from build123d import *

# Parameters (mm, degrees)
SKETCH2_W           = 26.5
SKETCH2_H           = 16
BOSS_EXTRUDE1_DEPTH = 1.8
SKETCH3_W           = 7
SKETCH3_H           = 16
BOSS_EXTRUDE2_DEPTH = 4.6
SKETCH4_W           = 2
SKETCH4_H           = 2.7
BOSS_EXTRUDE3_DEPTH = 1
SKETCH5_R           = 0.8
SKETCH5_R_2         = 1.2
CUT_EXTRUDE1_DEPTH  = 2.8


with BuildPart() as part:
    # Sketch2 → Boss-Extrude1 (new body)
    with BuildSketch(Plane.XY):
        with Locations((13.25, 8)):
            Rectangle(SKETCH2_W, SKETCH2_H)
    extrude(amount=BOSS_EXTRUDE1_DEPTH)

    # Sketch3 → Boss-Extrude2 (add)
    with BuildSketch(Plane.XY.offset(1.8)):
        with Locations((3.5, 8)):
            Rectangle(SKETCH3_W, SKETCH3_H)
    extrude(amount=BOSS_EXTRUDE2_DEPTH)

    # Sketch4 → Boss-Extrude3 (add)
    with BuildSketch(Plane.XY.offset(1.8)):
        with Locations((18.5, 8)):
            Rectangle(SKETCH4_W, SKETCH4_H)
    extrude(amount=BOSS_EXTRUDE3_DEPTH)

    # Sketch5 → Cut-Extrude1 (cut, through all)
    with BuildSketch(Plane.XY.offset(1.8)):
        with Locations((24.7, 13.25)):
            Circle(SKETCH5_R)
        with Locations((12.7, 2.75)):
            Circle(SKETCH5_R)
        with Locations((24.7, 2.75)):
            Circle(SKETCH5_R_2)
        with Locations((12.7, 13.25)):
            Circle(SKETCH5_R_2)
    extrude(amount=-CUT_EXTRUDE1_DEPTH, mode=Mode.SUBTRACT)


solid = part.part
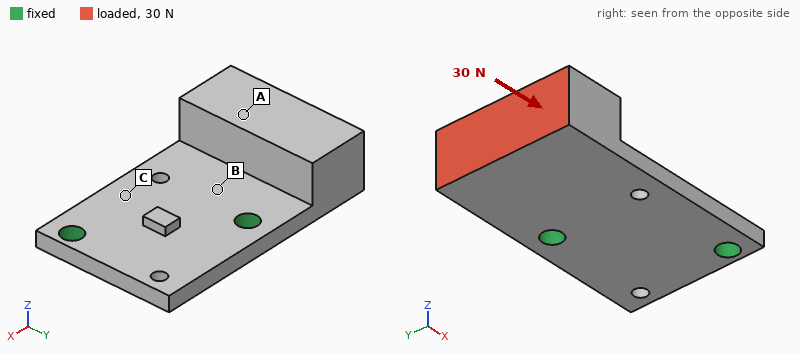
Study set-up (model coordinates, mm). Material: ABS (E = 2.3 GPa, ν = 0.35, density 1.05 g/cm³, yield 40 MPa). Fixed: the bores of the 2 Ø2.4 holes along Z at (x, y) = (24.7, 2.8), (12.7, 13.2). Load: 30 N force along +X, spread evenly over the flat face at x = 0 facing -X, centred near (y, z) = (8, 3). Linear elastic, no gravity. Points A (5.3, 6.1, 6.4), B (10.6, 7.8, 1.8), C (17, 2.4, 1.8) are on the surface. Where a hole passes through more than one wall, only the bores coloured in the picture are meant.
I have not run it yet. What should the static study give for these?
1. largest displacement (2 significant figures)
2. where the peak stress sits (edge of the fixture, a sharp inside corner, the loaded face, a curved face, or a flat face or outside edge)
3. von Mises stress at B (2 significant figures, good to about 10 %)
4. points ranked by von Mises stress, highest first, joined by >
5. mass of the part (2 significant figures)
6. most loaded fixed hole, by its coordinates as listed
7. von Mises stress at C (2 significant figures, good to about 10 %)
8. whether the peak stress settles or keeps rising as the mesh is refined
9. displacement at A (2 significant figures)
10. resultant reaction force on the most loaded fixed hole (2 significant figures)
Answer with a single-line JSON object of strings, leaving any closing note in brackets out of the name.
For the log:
{"largest displacement": "0.36 mm", "where the peak stress sits": "edge of the fixture", "von Mises stress at B": "7.2 MPa", "points ranked by von Mises stress, highest first, joined by >": "B > C > A", "mass of the part": "1.3 g", "most loaded fixed hole, by its coordinates as listed": "(12.7, 13.2)", "von Mises stress at C": "3.2 MPa", "whether the peak stress settles or keeps rising as the mesh is refined": "keeps rising", "displacement at A": "0.21 mm", "resultant reaction force on the most loaded fixed hole": "18 N"}
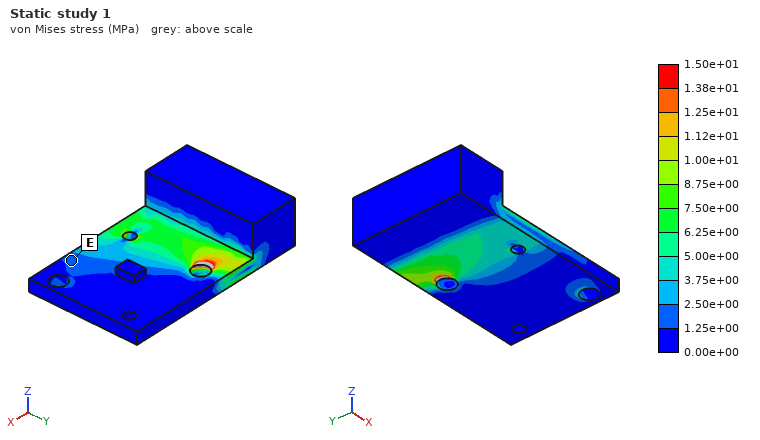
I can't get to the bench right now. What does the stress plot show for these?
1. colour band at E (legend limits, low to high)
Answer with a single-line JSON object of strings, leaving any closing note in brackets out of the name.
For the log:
{"colour band at E": "1.25e+00 to 2.50e+00 MPa"}
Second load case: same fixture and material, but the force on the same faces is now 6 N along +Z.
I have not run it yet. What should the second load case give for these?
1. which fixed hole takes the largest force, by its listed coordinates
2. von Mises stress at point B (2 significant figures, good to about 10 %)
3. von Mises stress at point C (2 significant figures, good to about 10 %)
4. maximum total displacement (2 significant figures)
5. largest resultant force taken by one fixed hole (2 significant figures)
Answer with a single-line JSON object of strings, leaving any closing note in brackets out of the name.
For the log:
{"which fixed hole takes the largest force, by its listed coordinates": "(12.7, 13.2)", "von Mises stress at point B": "5.8 MPa", "von Mises stress at point C": "2.8 MPa", "maximum total displacement": "0.38 mm", "largest resultant force taken by one fixed hole": "7.4 N"}
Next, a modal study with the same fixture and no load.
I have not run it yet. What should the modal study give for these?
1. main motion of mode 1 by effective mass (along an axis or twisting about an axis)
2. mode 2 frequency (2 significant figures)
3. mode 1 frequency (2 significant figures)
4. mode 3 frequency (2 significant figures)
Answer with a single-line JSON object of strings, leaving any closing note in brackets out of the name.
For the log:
{"main motion of mode 1 by effective mass": "along Z", "mode 2 frequency": "2400 Hz", "mode 1 frequency": "1100 Hz", "mode 3 frequency": "5100 Hz"}
